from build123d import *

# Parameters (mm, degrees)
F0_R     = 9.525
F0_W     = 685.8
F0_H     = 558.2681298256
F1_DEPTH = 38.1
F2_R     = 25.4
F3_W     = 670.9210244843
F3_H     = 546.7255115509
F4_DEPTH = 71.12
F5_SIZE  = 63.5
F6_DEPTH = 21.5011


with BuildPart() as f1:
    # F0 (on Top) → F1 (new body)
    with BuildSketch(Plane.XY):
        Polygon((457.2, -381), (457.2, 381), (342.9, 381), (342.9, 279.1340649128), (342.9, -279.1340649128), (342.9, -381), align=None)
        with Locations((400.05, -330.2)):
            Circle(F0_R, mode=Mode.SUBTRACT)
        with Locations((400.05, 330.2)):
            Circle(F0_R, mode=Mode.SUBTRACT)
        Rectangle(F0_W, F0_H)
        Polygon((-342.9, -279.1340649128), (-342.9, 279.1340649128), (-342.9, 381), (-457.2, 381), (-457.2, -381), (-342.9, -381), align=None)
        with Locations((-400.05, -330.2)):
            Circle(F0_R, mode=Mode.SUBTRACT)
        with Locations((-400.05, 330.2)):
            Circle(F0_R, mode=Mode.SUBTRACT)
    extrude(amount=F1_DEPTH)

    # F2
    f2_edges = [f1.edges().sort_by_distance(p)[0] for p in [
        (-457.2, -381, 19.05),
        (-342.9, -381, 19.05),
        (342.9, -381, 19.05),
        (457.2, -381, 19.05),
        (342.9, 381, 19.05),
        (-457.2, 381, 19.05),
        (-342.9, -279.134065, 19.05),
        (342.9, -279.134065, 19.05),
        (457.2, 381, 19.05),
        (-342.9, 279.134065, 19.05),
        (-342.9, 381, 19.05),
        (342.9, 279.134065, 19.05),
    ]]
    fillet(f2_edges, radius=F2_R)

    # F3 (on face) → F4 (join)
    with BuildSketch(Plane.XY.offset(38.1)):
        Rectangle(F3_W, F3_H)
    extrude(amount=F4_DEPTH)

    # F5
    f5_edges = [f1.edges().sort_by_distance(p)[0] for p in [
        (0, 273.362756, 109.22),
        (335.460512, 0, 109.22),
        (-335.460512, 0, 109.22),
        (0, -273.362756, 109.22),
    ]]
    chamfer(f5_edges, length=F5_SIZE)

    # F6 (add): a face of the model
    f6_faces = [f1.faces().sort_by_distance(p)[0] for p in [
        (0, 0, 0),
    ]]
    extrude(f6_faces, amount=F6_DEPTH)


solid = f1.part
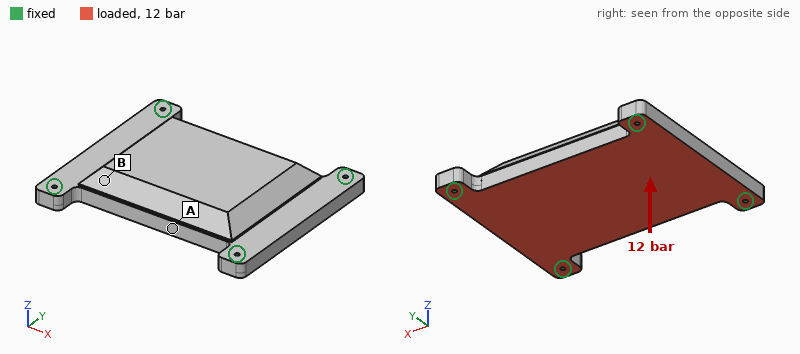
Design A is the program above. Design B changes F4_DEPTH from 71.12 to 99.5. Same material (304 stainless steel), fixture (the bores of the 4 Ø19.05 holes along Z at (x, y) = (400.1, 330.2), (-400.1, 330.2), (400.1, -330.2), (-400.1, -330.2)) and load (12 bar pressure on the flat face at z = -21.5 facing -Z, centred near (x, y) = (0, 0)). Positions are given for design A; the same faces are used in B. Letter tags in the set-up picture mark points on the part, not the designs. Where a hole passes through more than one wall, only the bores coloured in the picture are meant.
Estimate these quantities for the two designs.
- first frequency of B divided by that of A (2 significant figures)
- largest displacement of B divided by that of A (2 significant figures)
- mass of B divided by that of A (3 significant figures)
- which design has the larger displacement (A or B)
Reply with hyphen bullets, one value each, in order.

- 1.0
- 0.75
- 1.19
- A
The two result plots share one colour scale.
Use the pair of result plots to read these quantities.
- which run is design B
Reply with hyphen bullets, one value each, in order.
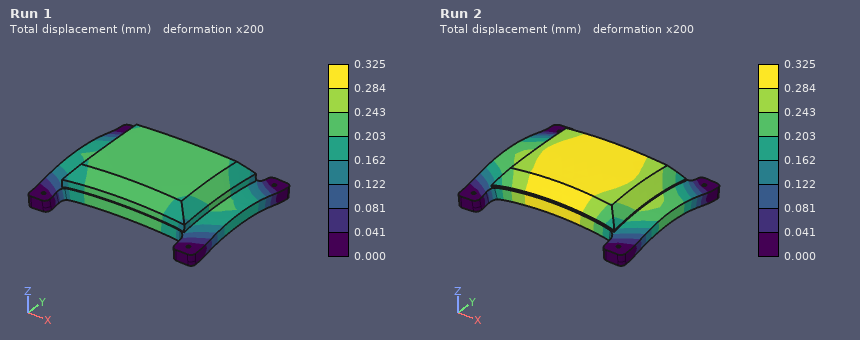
- Run 1
